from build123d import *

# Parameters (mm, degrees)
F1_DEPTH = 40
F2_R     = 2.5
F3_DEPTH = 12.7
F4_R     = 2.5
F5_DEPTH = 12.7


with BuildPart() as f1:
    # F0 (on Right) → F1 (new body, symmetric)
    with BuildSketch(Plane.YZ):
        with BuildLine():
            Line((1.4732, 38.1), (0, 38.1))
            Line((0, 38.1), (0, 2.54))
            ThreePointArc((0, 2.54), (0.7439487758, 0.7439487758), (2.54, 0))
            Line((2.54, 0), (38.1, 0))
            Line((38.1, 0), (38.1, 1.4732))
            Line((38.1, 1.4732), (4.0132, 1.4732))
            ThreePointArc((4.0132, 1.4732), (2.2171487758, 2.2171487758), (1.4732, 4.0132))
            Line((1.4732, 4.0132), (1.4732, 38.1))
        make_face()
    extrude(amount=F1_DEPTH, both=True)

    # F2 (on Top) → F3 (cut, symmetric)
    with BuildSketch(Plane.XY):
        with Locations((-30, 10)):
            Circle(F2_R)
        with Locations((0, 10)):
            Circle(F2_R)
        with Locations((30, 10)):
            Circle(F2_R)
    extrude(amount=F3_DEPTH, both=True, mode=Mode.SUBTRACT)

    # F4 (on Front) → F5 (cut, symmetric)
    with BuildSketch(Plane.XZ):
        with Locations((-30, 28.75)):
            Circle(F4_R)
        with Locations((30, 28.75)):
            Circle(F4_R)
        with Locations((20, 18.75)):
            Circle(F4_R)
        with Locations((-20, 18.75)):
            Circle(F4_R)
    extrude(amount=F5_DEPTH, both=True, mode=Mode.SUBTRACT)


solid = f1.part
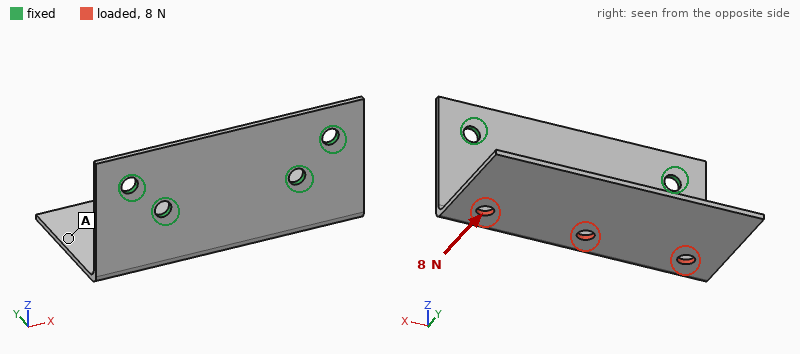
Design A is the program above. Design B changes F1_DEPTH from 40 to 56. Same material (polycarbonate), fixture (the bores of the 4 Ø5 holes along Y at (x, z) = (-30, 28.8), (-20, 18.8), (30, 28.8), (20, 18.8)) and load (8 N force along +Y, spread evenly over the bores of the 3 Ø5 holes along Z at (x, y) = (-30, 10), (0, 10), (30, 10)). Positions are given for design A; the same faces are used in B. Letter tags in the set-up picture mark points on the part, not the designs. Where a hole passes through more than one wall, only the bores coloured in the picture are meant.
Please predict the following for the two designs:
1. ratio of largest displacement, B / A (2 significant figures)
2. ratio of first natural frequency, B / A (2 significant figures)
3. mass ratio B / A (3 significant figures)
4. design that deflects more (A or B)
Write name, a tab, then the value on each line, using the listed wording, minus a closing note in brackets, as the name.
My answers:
ratio of largest displacement, B / A	0.85
ratio of first natural frequency, B / A	0.97
mass ratio B / A	1.41
design that deflects more	A
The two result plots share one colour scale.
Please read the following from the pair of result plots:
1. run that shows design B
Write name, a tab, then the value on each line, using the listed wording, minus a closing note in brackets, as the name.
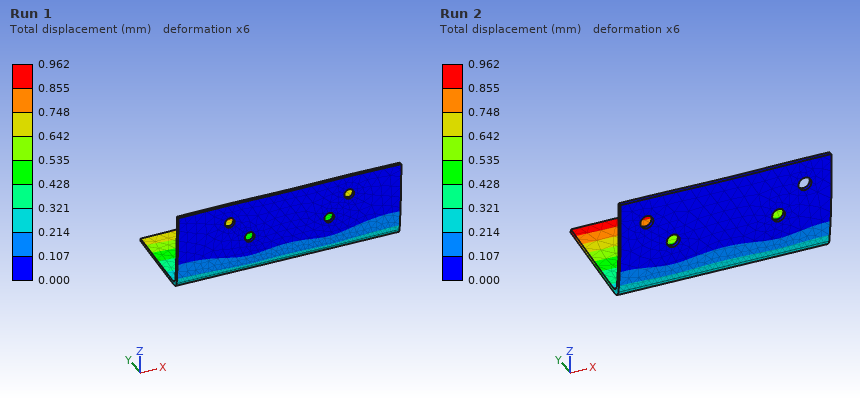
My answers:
run that shows design B	Run 1
